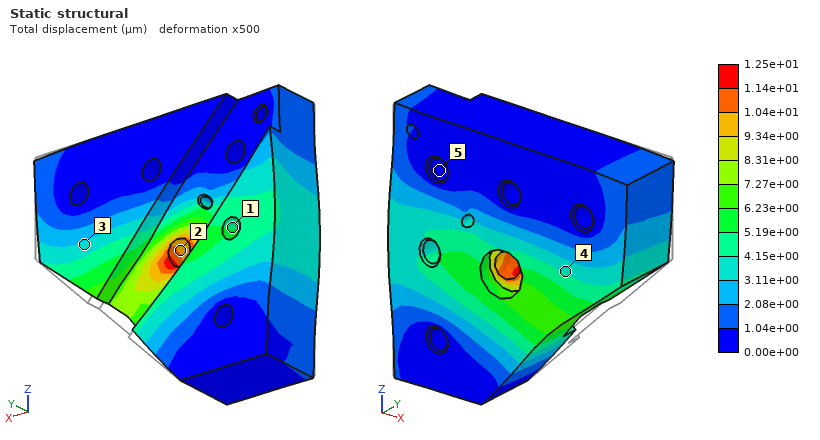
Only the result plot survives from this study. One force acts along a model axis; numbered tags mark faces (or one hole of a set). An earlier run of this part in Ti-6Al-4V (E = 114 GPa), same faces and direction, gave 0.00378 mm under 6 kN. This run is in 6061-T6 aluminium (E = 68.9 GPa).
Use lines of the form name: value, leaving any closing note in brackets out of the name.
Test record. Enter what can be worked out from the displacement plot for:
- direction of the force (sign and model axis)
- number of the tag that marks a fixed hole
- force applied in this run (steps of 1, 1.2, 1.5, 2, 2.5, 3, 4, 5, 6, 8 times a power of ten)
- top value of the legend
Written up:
direction of the force: -X
number of the tag that marks a fixed hole: 5
force applied in this run: 12 kN
top value of the legend: 1.25e+01 µm
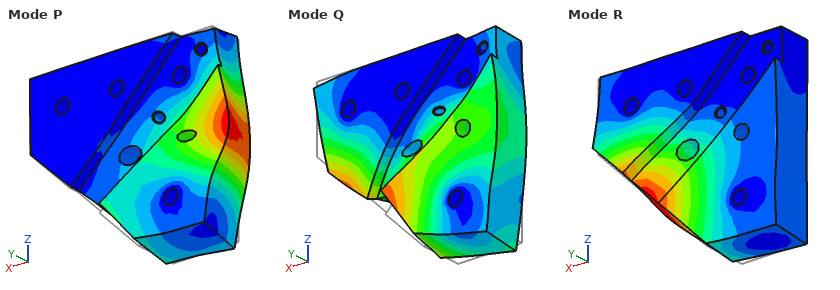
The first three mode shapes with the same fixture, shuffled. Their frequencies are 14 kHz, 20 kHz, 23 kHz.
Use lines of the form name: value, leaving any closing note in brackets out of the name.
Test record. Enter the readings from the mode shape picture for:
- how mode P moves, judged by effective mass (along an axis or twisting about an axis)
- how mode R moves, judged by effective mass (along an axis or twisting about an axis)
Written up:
how mode P moves, judged by effective mass: along Y
how mode R moves, judged by effective mass: along Y
